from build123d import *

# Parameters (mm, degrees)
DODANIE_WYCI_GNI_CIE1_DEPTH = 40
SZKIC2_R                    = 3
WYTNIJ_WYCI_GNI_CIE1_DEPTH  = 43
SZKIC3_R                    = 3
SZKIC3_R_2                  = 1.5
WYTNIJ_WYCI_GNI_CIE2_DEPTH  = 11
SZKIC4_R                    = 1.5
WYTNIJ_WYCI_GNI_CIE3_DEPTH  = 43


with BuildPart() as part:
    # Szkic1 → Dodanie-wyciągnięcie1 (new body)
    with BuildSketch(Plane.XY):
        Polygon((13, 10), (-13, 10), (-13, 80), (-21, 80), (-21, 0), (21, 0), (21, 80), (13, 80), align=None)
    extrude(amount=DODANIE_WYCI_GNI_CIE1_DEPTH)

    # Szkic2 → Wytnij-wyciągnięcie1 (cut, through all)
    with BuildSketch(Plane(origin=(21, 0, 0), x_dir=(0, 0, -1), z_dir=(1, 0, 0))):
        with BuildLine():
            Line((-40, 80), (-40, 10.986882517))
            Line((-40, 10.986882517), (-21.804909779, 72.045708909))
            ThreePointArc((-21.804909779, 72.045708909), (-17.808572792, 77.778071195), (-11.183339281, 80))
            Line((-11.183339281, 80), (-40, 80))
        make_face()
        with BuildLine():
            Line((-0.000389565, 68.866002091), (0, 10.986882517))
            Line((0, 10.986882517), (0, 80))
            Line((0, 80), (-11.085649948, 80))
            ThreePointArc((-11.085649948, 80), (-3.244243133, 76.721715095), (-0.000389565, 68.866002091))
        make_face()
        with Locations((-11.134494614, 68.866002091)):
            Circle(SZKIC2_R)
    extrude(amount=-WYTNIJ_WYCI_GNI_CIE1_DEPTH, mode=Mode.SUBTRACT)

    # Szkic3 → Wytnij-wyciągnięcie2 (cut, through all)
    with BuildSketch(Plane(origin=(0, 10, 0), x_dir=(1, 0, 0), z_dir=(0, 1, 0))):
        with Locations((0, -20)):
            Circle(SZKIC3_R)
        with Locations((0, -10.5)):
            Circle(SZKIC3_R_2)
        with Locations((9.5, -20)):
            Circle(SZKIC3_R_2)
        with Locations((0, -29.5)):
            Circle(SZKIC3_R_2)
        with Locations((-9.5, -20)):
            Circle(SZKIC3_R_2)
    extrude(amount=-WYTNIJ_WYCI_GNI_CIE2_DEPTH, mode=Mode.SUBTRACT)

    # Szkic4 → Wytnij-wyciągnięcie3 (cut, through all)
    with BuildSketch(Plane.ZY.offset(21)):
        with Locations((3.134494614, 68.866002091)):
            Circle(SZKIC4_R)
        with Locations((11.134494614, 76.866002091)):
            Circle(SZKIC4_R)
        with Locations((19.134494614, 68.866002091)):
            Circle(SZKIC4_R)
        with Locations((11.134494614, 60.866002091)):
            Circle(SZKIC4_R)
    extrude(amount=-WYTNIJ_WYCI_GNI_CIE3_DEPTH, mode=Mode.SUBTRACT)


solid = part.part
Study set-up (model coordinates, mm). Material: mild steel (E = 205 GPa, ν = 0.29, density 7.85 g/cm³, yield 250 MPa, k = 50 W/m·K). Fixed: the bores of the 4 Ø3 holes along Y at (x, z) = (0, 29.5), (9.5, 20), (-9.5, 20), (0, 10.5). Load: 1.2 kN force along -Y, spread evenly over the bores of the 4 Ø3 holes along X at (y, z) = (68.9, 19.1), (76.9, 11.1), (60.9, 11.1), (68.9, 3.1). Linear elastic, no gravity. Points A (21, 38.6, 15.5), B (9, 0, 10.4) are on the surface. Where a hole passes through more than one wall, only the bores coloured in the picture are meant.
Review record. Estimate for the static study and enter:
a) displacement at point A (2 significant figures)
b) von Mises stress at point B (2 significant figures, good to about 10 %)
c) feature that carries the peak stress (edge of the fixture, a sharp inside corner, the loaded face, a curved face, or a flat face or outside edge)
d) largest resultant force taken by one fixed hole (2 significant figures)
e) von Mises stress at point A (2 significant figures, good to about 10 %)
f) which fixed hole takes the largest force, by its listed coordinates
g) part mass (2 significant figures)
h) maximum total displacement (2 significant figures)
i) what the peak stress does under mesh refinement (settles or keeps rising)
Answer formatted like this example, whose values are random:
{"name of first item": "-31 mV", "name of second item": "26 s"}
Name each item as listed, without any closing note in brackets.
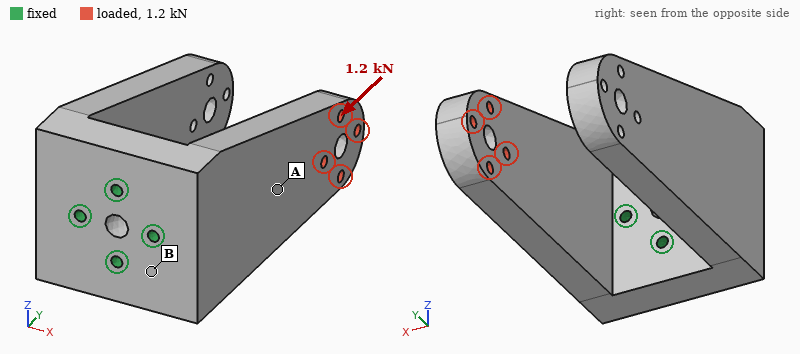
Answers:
{"displacement at point A": "6.7 µm", "von Mises stress at point B": "11 MPa", "feature that carries the peak stress": "edge of the fixture", "largest resultant force taken by one fixed hole": "1.1 kN", "von Mises stress at point A": "5.2 MPa", "which fixed hole takes the largest force, by its listed coordinates": "(9.5, 20)", "part mass": "380 g", "maximum total displacement": "16 µm", "what the peak stress does under mesh refinement": "keeps rising"}
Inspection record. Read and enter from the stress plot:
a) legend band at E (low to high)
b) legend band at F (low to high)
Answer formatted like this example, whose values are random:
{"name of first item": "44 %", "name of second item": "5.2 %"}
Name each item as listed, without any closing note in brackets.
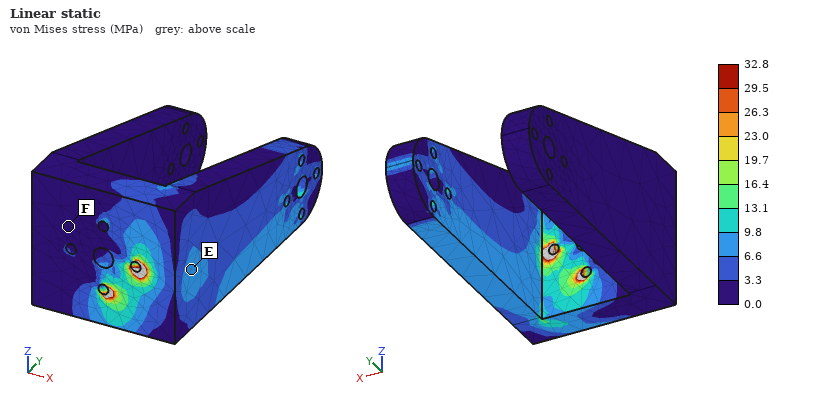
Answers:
{"legend band at E": "6.6 to 9.8 MPa", "legend band at F": "0.0 to 3.3 MPa"}
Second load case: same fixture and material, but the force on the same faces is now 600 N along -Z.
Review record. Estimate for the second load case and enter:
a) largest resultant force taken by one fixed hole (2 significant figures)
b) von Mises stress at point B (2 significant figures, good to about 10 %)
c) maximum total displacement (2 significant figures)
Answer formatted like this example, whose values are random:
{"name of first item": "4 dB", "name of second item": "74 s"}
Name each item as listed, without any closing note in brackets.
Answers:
{"largest resultant force taken by one fixed hole": "980 N", "von Mises stress at point B": "23 MPa", "maximum total displacement": "39 µm"}
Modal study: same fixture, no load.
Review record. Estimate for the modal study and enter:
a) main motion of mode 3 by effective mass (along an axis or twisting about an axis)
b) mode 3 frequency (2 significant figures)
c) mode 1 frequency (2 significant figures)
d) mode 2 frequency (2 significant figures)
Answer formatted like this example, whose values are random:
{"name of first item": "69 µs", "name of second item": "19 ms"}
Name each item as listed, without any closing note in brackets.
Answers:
{"main motion of mode 3 by effective mass": "twisting about Y", "mode 3 frequency": "3200 Hz", "mode 1 frequency": "1500 Hz", "mode 2 frequency": "1500 Hz"}
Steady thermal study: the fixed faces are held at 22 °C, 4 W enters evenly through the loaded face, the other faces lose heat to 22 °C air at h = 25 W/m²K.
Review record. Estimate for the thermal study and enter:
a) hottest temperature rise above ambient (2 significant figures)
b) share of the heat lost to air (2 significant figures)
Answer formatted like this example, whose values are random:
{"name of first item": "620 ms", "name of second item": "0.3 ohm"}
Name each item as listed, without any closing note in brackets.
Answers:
{"hottest temperature rise above ambient": "19 K", "share of the heat lost to air": "33 %"}
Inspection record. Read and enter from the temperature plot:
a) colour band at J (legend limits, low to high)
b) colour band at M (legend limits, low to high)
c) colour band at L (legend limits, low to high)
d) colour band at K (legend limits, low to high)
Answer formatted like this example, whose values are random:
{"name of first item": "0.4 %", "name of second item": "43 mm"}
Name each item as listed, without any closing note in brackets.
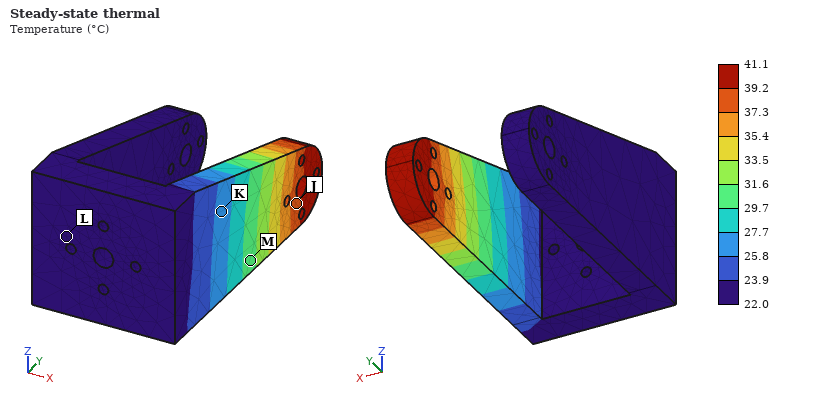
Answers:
{"colour band at J": "37.3 to 39.2 °C", "colour band at M": "29.7 to 31.6 °C", "colour band at L": "22.0 to 23.9 °C", "colour band at K": "25.8 to 27.7 °C"}
